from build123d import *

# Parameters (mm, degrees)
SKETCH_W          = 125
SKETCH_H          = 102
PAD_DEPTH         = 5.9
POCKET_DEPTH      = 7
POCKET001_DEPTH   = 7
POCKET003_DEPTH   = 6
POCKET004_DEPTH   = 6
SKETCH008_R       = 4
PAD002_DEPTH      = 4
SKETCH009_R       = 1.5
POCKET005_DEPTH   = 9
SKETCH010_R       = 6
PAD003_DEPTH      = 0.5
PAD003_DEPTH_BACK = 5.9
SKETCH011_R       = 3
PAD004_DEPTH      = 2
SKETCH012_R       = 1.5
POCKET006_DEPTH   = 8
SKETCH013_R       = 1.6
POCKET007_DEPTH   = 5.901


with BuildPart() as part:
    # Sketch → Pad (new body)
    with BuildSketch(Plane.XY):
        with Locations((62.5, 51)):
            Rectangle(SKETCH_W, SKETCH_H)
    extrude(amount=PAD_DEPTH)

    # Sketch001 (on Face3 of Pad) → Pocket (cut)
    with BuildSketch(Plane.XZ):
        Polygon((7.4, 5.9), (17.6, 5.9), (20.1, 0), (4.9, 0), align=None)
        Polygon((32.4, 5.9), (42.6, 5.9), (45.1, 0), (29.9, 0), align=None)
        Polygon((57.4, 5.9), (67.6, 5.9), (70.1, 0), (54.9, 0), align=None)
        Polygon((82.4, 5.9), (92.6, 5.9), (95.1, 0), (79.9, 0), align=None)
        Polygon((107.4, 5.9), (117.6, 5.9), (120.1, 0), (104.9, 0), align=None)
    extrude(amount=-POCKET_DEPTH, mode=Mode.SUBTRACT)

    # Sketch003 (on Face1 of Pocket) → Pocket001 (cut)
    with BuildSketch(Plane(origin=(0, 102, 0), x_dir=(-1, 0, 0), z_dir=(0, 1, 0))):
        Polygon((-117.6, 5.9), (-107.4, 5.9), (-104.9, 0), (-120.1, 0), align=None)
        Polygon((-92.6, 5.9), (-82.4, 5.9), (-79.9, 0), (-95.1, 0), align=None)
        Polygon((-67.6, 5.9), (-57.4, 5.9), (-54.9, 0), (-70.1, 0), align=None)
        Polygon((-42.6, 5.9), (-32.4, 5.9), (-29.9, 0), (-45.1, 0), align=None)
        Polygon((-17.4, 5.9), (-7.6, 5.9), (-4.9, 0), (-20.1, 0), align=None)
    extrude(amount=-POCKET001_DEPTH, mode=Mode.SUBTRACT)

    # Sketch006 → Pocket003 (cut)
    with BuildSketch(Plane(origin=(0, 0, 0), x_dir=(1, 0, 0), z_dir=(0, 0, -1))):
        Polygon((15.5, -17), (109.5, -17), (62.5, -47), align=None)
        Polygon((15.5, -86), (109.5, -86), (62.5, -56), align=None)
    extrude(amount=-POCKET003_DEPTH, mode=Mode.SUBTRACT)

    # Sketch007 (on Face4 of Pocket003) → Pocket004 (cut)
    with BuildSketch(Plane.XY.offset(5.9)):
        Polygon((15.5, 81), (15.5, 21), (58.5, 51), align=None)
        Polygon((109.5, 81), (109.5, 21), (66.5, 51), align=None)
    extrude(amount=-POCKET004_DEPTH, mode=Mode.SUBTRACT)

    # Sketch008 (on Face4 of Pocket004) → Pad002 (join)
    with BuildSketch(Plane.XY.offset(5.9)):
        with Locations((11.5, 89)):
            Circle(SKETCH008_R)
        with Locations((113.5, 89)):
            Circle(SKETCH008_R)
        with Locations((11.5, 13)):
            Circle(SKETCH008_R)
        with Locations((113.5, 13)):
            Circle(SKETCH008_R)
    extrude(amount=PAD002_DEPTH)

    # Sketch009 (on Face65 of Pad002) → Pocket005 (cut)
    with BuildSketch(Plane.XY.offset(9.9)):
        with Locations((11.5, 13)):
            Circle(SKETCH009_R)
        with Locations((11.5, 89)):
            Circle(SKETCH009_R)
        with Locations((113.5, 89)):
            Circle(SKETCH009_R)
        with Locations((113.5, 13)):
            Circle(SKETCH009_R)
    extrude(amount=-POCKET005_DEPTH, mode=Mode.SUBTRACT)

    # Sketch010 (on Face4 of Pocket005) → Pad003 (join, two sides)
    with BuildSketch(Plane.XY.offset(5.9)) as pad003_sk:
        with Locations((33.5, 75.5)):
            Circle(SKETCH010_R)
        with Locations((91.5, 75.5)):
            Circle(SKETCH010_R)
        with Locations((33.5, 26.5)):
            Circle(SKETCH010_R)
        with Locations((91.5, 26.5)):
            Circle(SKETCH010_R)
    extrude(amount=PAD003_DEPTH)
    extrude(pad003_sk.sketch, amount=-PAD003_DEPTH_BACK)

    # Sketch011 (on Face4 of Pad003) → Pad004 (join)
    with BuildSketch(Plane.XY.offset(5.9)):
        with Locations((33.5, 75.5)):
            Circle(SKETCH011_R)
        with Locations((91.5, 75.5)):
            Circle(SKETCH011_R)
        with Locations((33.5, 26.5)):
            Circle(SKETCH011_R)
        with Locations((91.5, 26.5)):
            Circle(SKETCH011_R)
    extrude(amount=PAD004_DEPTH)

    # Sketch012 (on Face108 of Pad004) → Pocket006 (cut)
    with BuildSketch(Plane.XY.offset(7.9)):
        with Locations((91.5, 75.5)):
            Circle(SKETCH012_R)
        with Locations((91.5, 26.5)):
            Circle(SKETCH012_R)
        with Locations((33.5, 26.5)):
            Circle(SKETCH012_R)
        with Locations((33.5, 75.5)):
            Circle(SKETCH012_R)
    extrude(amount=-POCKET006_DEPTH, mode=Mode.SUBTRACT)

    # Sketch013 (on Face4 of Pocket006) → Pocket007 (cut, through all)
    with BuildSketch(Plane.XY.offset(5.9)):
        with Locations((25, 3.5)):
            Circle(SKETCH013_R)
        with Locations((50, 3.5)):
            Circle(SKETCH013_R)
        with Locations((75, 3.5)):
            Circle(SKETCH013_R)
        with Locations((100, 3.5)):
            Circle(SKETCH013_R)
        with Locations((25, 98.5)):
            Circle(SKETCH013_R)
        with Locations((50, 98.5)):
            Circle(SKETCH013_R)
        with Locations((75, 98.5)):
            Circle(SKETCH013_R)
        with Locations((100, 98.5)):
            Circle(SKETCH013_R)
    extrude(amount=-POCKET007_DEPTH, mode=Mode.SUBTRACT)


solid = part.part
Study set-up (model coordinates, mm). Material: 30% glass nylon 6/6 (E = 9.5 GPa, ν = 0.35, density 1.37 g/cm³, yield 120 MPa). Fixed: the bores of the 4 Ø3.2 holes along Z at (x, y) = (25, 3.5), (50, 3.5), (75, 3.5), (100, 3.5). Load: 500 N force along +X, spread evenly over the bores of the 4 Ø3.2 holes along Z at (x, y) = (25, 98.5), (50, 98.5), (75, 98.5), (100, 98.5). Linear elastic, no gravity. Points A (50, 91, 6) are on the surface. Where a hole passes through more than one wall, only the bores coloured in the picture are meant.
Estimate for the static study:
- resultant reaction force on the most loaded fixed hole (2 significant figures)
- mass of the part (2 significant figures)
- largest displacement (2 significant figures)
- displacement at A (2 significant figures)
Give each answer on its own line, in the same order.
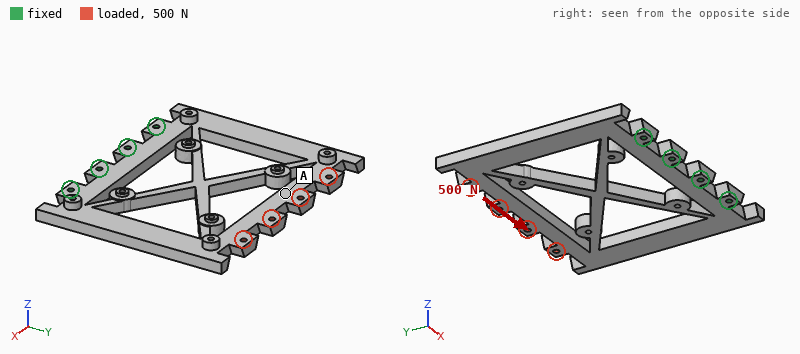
630 N
55 g
0.52 mm
0.46 mm
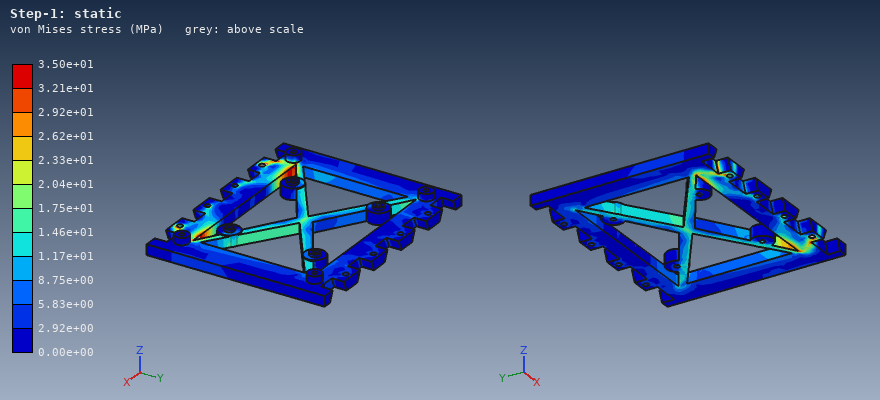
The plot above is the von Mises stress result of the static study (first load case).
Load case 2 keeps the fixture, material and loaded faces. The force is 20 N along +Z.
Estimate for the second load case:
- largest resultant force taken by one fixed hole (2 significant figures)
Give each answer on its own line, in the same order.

11 N
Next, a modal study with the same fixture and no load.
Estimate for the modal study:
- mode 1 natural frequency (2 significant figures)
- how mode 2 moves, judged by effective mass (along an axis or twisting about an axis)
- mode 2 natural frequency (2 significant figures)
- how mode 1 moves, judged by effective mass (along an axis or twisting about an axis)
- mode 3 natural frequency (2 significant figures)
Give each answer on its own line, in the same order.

140 Hz
twisting about Y
310 Hz
along Z
840 Hz
